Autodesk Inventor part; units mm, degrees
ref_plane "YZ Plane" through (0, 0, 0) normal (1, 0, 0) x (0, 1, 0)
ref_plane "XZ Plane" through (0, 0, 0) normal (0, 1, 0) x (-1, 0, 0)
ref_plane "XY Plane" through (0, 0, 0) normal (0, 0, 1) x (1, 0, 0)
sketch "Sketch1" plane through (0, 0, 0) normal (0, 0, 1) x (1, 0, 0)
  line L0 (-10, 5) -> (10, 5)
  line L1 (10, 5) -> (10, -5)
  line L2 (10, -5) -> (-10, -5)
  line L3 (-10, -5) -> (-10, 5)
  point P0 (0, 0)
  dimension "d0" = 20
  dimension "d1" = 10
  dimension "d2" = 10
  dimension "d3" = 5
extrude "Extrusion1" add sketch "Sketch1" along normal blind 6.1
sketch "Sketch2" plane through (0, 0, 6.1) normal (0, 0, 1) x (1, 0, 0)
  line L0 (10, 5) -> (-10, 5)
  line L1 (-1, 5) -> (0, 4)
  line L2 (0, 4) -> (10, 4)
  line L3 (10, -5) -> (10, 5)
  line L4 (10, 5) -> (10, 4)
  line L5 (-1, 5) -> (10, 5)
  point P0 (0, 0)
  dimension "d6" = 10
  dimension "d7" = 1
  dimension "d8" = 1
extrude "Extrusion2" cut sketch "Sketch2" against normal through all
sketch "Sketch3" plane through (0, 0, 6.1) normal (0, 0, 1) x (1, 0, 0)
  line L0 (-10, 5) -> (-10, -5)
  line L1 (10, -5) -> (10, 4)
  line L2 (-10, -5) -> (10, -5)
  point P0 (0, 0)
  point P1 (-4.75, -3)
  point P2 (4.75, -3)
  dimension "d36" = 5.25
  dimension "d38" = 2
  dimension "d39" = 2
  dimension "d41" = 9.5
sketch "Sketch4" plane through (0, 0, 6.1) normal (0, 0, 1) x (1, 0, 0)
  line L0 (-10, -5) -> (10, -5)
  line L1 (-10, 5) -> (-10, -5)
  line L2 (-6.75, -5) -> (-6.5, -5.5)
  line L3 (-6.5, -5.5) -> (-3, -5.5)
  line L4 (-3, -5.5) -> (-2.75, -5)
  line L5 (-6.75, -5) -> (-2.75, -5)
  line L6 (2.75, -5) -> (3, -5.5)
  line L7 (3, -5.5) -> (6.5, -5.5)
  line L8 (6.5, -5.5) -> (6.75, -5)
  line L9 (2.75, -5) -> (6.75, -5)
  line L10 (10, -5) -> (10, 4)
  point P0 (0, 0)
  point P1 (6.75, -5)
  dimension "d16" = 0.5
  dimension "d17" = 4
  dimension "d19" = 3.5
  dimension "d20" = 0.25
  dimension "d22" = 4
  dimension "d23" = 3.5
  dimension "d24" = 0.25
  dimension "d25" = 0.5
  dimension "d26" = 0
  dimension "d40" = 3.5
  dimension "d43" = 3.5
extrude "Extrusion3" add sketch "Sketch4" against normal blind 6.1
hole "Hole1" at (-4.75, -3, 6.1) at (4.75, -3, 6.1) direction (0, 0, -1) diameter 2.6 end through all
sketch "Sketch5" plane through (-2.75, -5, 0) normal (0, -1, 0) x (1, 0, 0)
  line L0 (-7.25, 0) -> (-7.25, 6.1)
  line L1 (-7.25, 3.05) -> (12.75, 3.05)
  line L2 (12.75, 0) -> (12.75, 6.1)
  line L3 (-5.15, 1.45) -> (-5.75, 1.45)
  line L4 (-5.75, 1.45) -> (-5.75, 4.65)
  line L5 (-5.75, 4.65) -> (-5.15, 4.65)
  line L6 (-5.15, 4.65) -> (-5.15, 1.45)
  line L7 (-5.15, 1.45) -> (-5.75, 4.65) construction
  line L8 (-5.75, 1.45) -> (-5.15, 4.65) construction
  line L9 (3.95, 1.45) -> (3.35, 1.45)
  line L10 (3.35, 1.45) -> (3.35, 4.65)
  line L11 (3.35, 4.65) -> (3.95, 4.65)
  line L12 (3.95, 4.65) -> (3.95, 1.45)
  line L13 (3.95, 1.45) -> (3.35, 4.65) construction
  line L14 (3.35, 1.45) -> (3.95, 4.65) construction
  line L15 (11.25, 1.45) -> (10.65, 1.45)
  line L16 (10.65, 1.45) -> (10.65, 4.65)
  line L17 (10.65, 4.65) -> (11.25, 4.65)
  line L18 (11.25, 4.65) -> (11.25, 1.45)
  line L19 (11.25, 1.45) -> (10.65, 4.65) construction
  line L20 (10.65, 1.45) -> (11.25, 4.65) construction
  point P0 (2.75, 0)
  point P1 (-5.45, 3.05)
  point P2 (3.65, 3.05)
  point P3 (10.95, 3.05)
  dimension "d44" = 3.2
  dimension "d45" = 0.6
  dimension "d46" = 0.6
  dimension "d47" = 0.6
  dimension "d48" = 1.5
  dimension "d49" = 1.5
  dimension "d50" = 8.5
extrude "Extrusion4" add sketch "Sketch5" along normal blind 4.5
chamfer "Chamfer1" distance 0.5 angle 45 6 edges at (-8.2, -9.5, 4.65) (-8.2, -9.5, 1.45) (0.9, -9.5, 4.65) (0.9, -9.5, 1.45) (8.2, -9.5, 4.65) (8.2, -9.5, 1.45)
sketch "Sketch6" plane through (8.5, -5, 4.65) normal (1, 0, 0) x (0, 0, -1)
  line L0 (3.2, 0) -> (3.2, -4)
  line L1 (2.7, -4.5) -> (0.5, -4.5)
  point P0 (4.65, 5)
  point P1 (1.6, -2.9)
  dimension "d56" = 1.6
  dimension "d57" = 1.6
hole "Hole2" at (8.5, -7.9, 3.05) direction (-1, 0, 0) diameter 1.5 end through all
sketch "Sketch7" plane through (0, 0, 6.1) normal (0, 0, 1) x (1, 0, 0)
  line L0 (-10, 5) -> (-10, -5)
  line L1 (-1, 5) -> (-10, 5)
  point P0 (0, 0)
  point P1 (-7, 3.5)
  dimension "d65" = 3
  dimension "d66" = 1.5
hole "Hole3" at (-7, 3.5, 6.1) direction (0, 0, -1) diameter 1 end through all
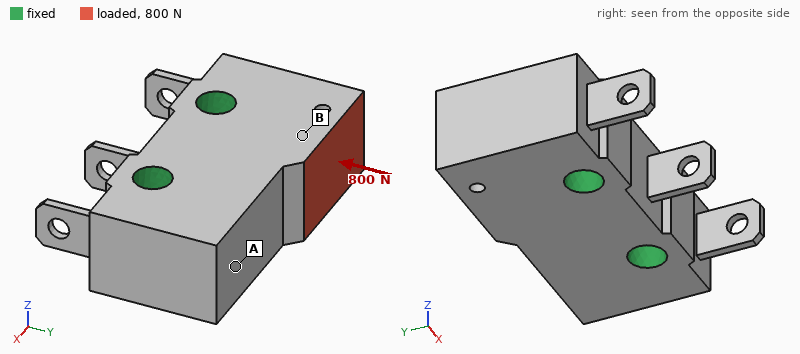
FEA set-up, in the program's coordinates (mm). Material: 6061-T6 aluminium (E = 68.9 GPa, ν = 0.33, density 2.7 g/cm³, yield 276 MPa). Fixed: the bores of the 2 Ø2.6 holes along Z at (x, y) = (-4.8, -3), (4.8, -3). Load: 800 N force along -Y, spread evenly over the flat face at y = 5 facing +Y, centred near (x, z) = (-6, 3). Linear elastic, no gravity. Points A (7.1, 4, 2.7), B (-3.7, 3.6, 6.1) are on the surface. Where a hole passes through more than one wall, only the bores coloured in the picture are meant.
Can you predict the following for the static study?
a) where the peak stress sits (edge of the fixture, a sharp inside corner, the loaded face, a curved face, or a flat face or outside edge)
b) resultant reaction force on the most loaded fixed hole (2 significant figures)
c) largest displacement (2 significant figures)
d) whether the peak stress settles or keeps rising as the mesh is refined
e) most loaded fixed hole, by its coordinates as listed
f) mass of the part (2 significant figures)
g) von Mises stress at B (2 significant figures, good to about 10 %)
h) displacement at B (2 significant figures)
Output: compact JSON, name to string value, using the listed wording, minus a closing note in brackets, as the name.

{"where the peak stress sits": "edge of the fixture", "resultant reaction force on the most loaded fixed hole": "790 N", "largest displacement": "3.6 µm", "whether the peak stress settles or keeps rising as the mesh is refined": "keeps rising", "most loaded fixed hole, by its coordinates as listed": "(-4.8, -3)", "mass of the part": "3.1 g", "von Mises stress at B": "16 MPa", "displacement at B": "1.7 µm"}
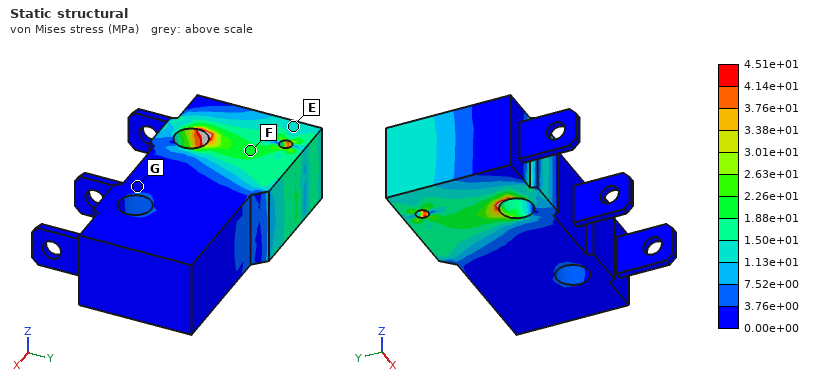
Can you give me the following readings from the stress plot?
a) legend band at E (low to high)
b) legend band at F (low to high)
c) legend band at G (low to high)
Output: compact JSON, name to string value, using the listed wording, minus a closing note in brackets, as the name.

{"legend band at E": "1.13e+01 to 1.50e+01 MPa", "legend band at F": "1.88e+01 to 2.26e+01 MPa", "legend band at G": "0.00e+00 to 3.76e+00 MPa"}
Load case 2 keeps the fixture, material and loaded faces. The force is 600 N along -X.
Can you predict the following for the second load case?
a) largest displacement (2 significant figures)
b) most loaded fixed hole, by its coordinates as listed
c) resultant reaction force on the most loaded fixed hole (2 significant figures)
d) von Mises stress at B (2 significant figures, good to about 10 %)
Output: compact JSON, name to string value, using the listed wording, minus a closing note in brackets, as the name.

{"largest displacement": "7.1 µm", "most loaded fixed hole, by its coordinates as listed": "(4.8, -3)", "resultant reaction force on the most loaded fixed hole": "520 N", "von Mises stress at B": "25 MPa"}
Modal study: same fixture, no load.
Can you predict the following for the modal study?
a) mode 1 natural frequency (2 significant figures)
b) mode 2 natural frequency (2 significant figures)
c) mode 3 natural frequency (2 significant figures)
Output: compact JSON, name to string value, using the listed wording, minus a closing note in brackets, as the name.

{"mode 1 natural frequency": "25 kHz", "mode 2 natural frequency": "25 kHz", "mode 3 natural frequency": "25 kHz"}
